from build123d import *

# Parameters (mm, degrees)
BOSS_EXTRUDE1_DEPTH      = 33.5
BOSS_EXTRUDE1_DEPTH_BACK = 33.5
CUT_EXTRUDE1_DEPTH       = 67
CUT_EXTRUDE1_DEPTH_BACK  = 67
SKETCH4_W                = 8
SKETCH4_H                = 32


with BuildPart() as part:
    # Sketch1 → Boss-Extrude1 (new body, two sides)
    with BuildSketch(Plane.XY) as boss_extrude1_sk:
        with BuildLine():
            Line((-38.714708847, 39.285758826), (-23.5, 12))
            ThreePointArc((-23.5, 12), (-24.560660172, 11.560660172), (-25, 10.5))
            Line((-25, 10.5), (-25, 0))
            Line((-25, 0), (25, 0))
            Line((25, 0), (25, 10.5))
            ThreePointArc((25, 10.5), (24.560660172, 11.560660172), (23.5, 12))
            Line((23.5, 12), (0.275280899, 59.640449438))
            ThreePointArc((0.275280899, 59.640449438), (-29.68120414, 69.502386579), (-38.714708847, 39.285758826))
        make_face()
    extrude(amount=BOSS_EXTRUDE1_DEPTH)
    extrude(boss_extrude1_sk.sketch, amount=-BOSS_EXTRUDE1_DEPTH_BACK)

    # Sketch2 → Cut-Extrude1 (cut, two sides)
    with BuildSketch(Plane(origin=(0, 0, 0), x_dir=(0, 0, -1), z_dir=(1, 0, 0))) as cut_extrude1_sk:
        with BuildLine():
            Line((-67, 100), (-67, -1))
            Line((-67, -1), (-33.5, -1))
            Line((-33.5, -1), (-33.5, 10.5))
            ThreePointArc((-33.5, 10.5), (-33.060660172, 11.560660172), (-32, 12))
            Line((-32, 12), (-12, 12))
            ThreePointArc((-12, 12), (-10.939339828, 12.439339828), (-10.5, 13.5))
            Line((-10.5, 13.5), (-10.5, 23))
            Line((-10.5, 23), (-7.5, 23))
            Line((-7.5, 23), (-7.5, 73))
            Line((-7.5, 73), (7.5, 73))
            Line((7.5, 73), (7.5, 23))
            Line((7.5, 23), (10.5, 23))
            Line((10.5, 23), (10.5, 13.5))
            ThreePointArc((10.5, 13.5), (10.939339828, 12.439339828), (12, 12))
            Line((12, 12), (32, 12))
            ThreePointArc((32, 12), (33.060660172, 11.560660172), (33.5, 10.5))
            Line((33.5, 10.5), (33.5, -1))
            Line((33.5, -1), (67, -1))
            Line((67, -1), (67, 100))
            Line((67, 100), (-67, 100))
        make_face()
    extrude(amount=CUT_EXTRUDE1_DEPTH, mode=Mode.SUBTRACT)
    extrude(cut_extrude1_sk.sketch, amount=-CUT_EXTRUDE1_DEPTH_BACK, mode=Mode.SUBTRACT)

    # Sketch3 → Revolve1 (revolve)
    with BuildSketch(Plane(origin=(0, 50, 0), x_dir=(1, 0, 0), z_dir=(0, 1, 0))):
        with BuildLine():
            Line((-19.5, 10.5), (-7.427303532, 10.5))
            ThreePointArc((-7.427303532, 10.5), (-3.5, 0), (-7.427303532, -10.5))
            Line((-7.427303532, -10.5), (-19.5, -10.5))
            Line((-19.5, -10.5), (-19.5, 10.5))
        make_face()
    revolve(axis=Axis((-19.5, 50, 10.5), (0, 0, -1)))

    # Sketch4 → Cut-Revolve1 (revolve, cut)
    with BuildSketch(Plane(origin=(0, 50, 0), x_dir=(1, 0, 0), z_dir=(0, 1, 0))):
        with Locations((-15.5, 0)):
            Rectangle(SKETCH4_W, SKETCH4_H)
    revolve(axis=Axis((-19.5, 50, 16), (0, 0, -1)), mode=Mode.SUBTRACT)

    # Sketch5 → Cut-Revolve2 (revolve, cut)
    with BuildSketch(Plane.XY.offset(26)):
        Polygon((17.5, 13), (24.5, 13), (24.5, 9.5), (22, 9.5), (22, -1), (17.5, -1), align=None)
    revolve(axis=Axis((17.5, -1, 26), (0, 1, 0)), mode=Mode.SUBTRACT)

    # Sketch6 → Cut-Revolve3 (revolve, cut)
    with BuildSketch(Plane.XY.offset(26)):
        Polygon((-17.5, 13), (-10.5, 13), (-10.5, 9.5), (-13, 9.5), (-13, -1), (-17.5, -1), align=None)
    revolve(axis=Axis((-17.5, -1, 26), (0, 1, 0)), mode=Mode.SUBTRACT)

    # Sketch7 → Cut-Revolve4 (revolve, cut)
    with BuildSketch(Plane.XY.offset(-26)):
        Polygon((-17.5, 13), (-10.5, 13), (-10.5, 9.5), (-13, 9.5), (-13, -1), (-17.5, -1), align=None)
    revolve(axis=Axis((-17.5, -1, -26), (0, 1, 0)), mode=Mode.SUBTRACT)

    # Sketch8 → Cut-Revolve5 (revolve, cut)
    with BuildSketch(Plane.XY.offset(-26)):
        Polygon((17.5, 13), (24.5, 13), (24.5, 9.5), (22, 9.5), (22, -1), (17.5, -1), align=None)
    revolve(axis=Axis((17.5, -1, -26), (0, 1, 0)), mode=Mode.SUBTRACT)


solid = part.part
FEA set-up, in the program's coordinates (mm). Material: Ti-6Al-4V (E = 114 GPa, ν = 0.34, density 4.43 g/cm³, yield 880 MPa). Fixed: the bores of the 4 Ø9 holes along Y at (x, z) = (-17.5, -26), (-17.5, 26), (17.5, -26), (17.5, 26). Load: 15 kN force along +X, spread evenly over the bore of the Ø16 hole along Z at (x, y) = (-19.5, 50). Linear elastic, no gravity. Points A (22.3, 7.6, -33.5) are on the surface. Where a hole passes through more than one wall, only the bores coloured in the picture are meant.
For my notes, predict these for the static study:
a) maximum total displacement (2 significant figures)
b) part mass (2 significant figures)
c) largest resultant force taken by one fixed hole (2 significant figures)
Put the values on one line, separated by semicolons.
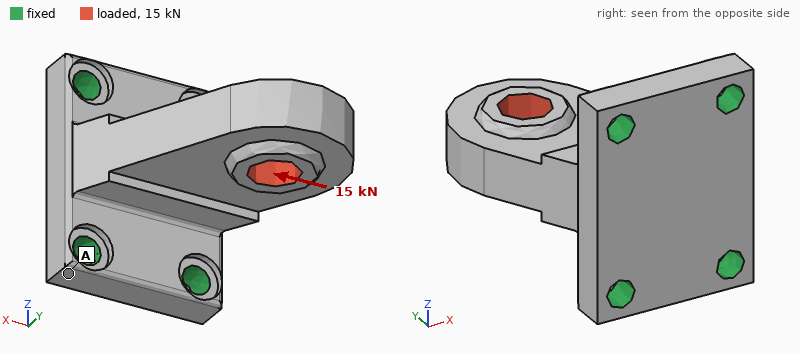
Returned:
0.20 mm; 340 g; 11 kN
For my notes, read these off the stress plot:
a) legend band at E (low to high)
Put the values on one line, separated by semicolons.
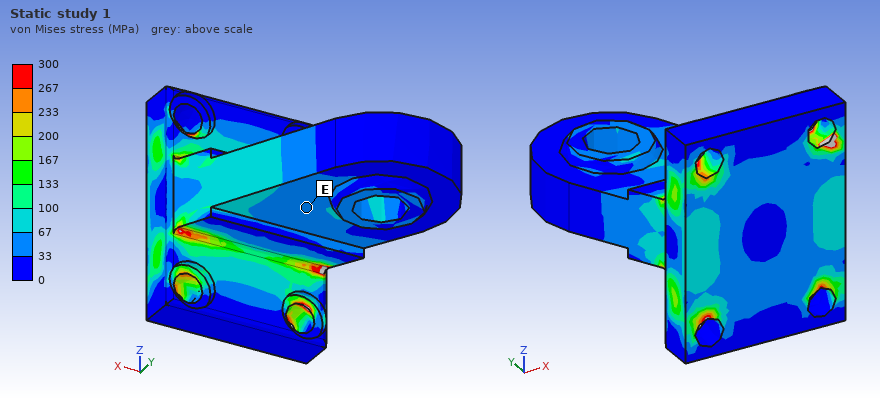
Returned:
33 to 67 MPa
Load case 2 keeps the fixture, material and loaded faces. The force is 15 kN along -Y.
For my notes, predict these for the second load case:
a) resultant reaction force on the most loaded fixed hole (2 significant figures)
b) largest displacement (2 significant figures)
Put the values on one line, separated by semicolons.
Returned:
8.5 kN; 90 µm
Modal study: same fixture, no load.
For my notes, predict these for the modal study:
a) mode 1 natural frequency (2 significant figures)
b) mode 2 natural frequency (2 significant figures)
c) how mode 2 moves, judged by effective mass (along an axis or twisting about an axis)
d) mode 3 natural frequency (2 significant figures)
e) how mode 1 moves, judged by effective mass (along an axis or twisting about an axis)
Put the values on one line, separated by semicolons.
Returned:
3600 Hz; 4500 Hz; along X; 9300 Hz; along Z
